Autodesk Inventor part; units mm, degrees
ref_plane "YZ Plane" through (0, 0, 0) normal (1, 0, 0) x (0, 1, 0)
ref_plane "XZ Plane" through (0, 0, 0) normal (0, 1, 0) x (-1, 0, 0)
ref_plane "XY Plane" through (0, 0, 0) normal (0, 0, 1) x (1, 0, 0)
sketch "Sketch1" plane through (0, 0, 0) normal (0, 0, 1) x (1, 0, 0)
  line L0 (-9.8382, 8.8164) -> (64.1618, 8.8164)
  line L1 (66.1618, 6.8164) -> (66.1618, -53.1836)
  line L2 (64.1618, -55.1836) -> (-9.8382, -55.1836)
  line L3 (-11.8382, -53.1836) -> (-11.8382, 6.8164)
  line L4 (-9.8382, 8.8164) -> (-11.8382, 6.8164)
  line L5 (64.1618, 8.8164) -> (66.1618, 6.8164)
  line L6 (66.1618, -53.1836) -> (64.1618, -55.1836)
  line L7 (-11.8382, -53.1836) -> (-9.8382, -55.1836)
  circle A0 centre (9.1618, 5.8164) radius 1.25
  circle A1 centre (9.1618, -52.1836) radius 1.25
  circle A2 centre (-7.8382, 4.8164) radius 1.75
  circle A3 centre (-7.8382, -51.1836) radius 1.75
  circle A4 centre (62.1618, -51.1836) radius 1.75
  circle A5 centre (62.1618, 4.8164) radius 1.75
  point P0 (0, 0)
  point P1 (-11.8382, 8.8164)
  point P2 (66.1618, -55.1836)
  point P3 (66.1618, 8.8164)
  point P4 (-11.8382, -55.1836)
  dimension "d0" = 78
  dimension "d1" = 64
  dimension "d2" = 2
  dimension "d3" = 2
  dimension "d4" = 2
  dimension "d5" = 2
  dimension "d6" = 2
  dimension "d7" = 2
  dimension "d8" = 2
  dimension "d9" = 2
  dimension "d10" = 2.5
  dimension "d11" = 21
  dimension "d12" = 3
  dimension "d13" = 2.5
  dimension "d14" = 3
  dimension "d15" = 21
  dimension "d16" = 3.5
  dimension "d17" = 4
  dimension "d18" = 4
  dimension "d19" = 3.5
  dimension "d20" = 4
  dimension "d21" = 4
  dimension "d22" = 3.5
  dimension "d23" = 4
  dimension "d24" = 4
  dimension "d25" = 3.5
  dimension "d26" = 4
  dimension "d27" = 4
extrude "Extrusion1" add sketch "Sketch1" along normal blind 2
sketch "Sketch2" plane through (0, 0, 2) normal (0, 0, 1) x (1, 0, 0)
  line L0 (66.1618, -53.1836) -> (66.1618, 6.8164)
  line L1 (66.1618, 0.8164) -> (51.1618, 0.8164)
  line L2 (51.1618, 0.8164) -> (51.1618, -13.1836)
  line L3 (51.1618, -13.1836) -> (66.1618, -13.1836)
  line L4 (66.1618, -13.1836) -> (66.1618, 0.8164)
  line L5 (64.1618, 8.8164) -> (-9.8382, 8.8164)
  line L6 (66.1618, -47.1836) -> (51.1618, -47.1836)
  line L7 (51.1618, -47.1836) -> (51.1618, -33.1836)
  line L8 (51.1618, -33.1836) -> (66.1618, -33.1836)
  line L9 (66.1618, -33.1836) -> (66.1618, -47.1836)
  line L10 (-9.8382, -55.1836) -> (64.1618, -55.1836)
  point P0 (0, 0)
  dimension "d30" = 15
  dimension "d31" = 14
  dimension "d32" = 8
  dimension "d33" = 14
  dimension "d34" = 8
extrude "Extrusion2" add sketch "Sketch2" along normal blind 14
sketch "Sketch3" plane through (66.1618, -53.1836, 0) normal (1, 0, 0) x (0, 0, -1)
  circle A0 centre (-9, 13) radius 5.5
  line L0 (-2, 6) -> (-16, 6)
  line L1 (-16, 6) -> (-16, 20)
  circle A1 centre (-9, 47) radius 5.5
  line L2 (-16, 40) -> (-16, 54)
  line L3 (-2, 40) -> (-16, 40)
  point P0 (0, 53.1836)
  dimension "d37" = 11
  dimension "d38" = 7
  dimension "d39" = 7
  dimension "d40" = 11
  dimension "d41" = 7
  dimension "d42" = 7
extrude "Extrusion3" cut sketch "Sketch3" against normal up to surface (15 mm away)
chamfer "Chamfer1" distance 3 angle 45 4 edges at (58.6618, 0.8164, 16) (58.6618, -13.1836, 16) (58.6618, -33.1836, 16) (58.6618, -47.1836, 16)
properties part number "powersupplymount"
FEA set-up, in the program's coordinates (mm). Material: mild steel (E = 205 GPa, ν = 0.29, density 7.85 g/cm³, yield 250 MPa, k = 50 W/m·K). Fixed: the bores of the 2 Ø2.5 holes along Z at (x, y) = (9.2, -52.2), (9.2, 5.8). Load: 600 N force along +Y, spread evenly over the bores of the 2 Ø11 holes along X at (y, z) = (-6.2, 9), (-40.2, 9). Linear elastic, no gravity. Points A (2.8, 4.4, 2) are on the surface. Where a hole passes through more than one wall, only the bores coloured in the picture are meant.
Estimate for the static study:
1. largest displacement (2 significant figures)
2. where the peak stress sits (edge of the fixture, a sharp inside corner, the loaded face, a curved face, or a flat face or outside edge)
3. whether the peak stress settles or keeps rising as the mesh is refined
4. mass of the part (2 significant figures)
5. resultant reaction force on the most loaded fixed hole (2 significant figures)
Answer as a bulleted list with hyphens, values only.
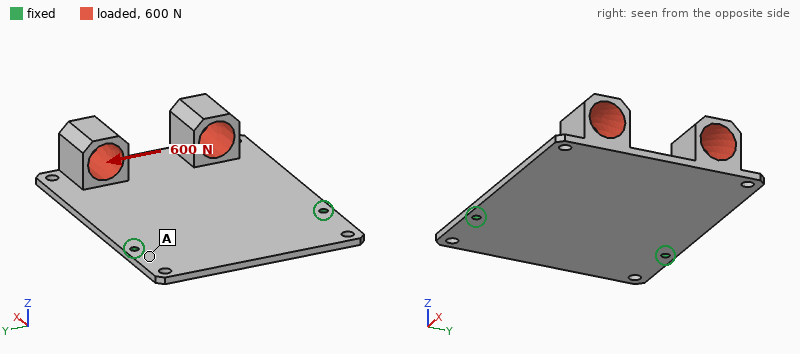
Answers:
- 0.29 mm
- edge of the fixture
- keeps rising
- 99 g
- 600 N
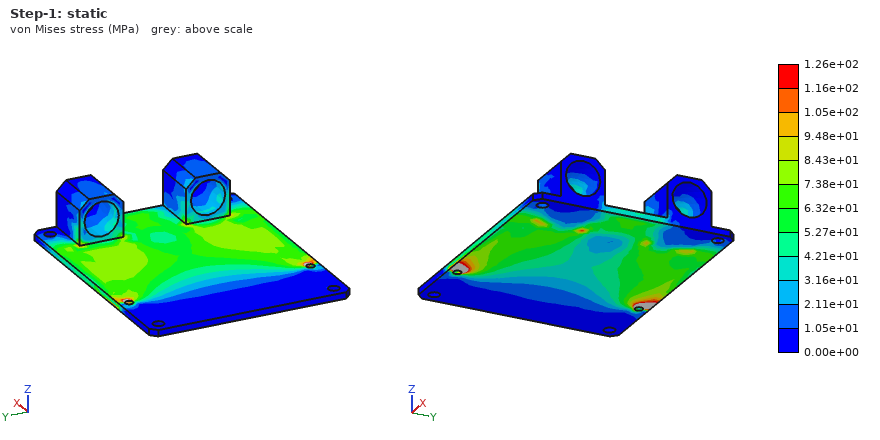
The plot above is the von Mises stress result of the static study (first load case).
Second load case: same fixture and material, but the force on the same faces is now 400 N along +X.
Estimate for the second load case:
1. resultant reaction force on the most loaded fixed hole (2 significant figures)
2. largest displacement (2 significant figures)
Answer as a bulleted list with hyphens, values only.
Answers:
- 200 N
- 0.77 mm
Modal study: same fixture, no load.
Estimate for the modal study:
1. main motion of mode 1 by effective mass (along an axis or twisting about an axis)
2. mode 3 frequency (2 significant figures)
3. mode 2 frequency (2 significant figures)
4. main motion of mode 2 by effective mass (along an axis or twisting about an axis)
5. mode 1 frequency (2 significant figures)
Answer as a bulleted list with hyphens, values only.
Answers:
- along Z
- 2000 Hz
- 900 Hz
- twisting about X
- 290 Hz
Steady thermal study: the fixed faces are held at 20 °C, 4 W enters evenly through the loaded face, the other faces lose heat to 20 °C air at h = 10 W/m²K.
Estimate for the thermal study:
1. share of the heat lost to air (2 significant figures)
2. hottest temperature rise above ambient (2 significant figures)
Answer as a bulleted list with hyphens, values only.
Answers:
- 42 %
- 29 K
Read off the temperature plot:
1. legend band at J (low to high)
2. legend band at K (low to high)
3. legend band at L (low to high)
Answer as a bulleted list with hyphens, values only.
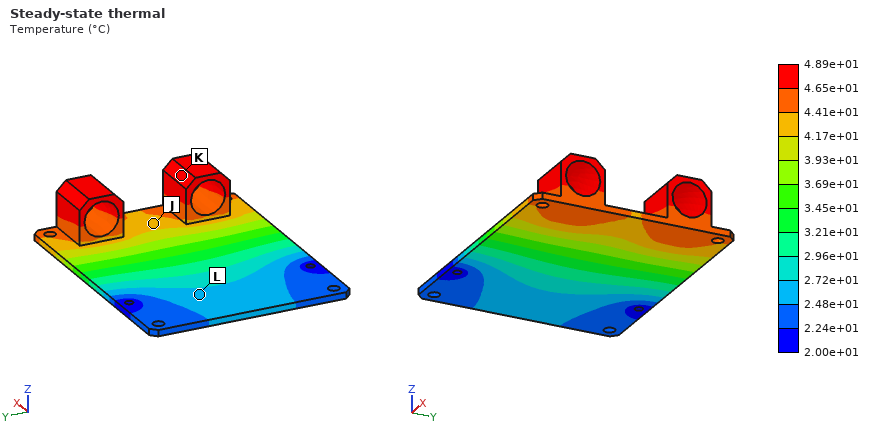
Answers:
- 4.17e+01 to 4.41e+01 °C
- 4.65e+01 to 4.89e+01 °C
- 2.48e+01 to 2.72e+01 °C
